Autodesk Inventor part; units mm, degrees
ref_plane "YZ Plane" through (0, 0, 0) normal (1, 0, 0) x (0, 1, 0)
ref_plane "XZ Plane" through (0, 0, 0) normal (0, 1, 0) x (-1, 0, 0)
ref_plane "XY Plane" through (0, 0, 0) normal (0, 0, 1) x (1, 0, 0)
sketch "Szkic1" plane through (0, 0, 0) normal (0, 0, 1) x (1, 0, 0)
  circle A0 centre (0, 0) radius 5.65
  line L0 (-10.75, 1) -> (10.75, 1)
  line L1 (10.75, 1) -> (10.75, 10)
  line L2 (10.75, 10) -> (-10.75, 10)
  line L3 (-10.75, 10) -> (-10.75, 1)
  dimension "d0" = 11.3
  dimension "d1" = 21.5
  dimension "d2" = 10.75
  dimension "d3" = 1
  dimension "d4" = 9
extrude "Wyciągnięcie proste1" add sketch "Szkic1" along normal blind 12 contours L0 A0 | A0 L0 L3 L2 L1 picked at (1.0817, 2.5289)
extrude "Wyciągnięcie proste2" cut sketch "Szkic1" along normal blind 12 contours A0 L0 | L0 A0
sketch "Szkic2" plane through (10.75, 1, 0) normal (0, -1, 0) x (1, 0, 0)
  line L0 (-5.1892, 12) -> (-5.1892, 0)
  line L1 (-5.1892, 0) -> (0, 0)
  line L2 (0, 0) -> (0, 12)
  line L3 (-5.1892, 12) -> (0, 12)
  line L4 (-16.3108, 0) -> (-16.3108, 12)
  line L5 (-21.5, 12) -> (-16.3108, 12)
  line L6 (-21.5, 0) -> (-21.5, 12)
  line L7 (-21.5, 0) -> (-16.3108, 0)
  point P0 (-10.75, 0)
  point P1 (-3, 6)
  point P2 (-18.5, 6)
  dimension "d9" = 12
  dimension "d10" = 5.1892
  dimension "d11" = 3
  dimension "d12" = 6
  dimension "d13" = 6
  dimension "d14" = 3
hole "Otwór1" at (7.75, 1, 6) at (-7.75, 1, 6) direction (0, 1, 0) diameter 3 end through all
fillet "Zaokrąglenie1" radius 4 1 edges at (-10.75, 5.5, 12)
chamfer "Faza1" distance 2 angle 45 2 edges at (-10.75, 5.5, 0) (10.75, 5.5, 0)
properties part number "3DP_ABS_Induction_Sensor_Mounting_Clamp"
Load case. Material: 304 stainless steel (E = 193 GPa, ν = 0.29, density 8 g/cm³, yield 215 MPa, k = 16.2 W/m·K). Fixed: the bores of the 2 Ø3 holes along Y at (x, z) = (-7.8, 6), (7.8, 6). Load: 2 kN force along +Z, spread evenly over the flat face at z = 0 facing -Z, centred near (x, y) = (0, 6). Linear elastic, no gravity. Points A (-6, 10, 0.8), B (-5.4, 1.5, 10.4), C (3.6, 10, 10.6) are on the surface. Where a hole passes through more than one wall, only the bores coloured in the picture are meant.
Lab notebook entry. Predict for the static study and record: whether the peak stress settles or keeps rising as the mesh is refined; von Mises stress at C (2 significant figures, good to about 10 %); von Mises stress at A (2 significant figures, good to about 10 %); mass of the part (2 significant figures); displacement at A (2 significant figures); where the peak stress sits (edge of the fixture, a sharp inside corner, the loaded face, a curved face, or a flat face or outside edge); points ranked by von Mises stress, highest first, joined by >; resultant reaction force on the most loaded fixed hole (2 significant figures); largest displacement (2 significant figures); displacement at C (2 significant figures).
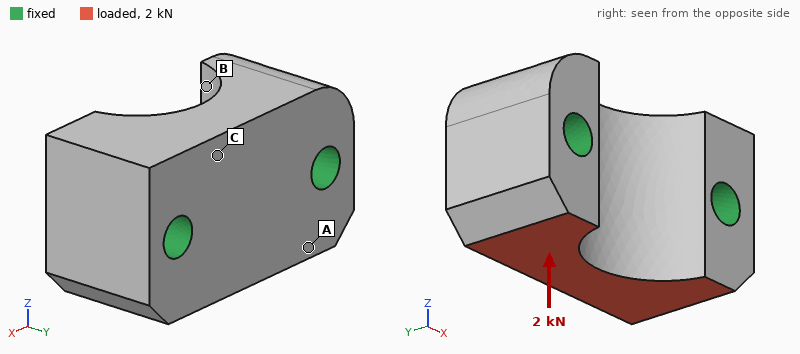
keeps rising
9.7 MPa
16 MPa
13 g
0.67 µm
edge of the fixture
A > C > B
1.0 kN
1.3 µm
0.52 µm
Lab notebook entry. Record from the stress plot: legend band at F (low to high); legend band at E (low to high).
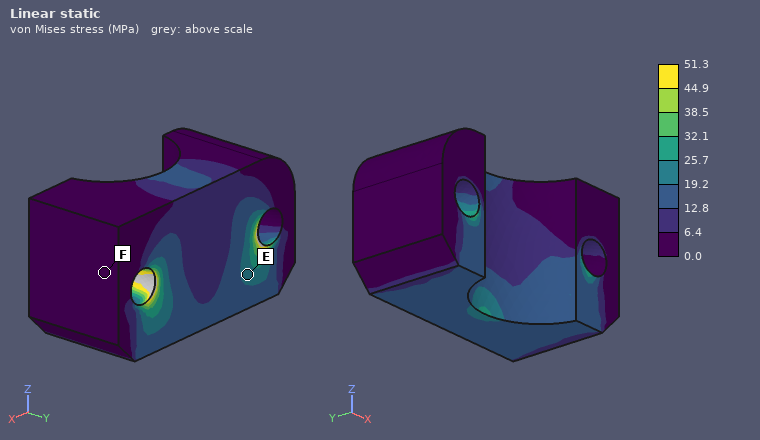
0.0 to 6.4 MPa
19.2 to 25.7 MPa
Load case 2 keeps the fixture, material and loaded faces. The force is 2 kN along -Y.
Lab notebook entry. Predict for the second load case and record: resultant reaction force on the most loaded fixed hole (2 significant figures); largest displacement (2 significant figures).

1.0 kN
4.2 µm
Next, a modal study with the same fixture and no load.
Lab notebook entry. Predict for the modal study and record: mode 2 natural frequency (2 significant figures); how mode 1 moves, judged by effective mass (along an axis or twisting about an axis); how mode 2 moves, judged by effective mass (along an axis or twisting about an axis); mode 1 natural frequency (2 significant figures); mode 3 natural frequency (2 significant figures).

83 kHz
along Z
along Y
78 kHz
96 kHz
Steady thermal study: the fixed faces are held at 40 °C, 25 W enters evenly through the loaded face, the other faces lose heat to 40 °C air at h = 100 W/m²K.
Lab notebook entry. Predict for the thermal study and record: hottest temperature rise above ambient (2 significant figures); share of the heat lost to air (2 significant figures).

81 K
5.7 %
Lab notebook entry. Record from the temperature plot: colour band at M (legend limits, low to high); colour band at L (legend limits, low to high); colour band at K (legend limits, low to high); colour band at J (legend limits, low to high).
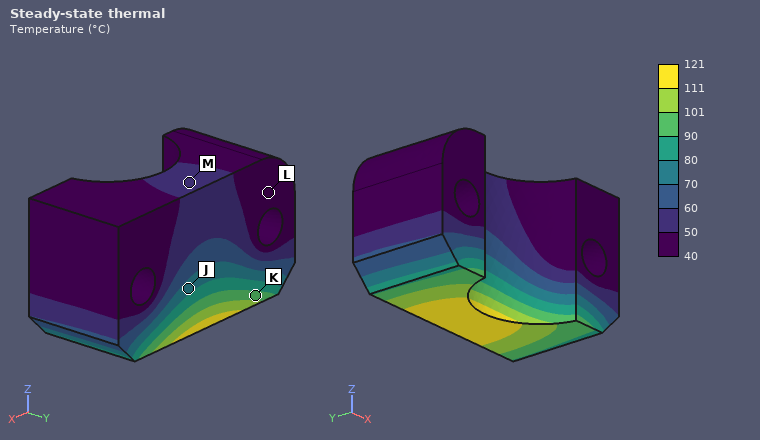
50 to 60 °C
40 to 50 °C
90 to 101 °C
70 to 80 °C
